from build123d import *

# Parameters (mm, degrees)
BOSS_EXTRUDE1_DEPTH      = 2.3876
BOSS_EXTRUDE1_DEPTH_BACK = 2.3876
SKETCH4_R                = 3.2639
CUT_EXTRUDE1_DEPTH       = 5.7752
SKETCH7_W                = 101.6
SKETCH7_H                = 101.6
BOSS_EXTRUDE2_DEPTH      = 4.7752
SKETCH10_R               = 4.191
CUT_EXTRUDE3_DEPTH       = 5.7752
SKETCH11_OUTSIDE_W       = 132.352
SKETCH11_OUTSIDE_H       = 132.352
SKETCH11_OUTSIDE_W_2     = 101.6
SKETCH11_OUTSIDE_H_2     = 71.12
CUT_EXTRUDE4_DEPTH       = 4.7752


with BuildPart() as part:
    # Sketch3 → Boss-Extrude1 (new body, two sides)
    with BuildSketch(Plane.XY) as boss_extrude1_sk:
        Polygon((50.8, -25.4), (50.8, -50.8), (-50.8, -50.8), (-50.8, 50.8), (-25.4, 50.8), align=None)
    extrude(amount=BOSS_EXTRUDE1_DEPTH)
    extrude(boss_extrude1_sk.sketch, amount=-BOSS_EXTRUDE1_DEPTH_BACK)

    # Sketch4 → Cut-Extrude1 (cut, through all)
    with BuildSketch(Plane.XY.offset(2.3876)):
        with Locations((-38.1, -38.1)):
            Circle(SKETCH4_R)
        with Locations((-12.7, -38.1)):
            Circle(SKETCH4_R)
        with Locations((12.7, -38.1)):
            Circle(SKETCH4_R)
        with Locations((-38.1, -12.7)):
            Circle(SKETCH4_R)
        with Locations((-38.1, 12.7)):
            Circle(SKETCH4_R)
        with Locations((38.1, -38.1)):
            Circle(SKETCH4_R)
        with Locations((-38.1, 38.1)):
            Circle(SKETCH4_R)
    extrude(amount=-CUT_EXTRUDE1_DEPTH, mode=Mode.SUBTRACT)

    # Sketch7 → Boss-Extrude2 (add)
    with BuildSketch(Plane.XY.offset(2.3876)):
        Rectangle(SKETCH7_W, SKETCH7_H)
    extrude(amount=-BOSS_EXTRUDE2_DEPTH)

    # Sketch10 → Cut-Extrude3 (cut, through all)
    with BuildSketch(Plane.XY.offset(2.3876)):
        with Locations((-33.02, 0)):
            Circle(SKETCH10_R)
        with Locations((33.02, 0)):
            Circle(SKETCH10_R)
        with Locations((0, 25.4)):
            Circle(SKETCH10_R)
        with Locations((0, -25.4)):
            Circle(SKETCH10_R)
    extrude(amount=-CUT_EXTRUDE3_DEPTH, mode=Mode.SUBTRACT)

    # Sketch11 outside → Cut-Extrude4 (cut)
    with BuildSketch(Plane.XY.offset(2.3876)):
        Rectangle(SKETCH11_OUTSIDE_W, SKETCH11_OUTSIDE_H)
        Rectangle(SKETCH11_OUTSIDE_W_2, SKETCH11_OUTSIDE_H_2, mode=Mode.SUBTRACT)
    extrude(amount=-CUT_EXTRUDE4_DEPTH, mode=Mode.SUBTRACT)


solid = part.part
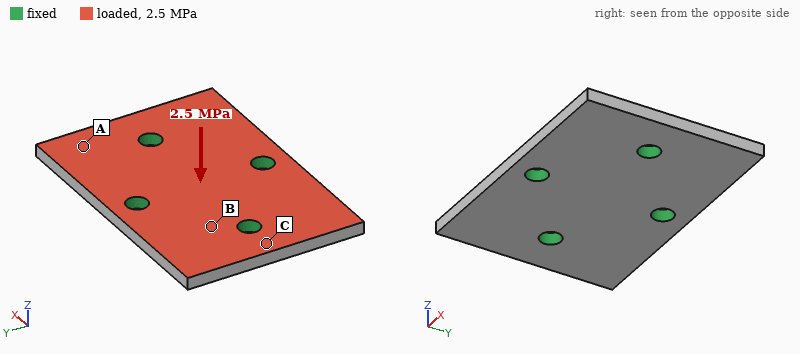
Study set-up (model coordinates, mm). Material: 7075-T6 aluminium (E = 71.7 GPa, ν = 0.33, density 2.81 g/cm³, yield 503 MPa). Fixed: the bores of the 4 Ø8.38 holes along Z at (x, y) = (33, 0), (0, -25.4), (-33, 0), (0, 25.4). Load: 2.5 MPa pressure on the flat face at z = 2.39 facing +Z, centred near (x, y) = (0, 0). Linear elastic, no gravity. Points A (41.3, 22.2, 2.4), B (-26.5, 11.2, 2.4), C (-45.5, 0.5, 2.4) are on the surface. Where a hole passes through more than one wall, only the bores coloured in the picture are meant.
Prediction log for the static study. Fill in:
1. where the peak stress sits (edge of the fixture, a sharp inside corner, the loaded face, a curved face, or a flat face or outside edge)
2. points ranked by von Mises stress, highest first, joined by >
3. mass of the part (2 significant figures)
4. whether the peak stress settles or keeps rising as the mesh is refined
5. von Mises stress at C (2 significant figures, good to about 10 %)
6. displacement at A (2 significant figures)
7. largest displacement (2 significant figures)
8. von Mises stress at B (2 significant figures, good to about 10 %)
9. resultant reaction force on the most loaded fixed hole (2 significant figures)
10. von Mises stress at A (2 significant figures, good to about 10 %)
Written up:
edge of the fixture
C > B > A
94 g
keeps rising
160 MPa
0.19 mm
0.41 mm
99 MPa
5.2 kN
40 MPa
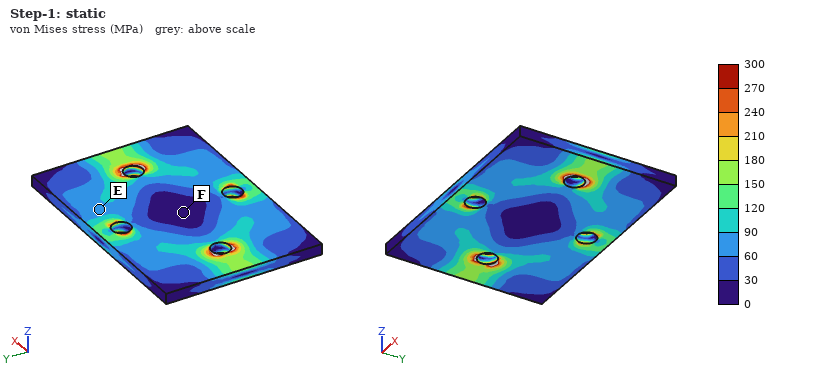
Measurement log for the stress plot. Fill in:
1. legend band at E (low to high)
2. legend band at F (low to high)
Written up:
60 to 90 MPa
0 to 30 MPa
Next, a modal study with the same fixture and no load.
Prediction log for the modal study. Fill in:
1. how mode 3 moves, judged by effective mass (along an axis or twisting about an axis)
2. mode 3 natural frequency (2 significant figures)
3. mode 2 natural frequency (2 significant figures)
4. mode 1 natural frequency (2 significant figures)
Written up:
along Z
4800 Hz
4500 Hz
4500 Hz
